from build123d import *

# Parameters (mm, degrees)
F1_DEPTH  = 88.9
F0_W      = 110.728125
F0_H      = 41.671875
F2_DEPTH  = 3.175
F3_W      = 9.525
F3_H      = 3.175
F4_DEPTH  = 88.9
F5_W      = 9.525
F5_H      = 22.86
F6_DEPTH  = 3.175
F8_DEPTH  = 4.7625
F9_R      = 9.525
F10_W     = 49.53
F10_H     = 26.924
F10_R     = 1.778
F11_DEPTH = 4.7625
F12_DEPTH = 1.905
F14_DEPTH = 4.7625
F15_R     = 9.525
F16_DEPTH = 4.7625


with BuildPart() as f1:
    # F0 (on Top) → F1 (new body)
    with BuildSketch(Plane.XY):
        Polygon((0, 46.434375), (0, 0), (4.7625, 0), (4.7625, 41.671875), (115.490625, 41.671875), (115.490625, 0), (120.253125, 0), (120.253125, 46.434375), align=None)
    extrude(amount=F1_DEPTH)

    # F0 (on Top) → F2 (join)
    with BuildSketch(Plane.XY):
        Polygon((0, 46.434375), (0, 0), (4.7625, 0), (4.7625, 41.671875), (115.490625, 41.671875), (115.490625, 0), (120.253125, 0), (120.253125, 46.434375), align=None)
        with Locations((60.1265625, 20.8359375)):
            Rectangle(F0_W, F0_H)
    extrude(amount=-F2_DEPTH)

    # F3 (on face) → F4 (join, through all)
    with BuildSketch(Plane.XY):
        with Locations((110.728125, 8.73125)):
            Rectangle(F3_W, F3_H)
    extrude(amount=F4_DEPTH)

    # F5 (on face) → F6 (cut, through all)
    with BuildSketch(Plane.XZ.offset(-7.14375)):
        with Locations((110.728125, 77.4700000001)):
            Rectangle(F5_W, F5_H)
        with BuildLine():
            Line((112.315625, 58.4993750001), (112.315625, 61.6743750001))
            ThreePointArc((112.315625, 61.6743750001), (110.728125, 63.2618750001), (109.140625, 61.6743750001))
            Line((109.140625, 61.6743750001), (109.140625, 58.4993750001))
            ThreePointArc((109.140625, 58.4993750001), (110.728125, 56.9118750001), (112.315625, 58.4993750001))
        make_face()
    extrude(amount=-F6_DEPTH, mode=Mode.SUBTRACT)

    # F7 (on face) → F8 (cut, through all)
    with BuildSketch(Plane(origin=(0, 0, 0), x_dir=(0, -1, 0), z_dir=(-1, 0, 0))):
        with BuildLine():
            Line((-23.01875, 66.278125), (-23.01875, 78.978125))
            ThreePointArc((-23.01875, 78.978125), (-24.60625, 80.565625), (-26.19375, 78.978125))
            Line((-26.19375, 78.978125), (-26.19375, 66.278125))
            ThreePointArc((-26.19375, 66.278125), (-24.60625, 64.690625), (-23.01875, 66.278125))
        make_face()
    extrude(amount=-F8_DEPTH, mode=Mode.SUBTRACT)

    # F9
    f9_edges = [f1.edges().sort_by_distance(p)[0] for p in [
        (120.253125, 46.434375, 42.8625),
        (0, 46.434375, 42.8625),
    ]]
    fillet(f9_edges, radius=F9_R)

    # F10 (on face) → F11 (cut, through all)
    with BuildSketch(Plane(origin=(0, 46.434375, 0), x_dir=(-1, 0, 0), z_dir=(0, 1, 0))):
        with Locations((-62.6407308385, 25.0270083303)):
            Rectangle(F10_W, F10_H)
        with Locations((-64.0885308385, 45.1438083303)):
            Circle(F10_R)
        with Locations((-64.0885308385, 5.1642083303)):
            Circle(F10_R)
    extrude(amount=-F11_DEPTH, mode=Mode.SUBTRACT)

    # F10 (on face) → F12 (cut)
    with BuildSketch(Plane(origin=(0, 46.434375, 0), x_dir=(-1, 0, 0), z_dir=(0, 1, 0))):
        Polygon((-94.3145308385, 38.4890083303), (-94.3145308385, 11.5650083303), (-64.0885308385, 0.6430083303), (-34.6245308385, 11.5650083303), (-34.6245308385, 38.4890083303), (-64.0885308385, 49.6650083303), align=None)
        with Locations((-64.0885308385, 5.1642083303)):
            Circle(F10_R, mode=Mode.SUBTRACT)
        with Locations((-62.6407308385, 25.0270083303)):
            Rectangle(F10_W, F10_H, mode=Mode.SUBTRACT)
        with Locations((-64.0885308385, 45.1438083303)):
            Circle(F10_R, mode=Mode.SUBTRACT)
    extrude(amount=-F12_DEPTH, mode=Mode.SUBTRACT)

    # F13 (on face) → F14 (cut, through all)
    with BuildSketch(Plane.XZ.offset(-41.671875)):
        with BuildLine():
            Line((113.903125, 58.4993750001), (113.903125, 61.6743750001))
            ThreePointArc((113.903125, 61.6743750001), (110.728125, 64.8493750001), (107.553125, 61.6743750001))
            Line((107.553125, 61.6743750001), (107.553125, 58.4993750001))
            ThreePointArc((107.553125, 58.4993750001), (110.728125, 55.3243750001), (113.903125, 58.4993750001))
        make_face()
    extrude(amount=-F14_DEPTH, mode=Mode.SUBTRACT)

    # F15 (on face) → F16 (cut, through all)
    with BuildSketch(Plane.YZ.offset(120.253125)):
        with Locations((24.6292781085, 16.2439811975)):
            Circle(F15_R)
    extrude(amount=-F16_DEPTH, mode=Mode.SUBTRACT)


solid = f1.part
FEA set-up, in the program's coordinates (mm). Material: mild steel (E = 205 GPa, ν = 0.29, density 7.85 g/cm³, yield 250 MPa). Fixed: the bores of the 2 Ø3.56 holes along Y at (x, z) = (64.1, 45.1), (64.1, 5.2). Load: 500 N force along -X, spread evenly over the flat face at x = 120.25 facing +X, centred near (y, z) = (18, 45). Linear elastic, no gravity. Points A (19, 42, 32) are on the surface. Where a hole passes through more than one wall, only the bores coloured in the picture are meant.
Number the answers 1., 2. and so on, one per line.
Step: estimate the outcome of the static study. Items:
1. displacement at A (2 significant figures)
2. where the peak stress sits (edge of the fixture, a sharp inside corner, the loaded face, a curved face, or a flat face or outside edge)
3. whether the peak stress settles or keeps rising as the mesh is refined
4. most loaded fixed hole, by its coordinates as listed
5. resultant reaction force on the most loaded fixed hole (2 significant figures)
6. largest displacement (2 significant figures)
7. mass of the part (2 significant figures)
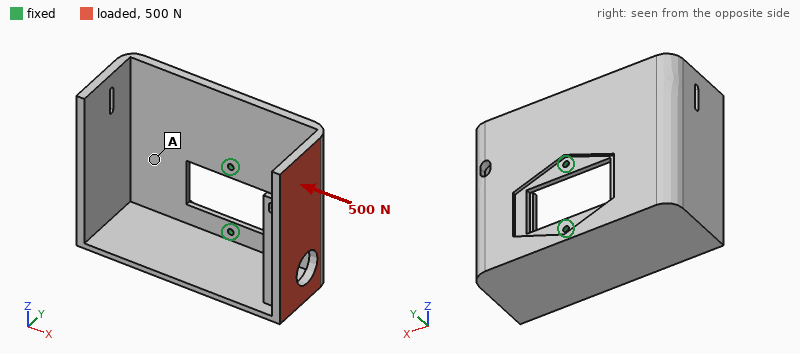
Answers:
1. 0.098 mm
2. edge of the fixture
3. keeps rising
4. (64.1, 45.1)
5. 490 N
6. 0.26 mm
7. 720 g
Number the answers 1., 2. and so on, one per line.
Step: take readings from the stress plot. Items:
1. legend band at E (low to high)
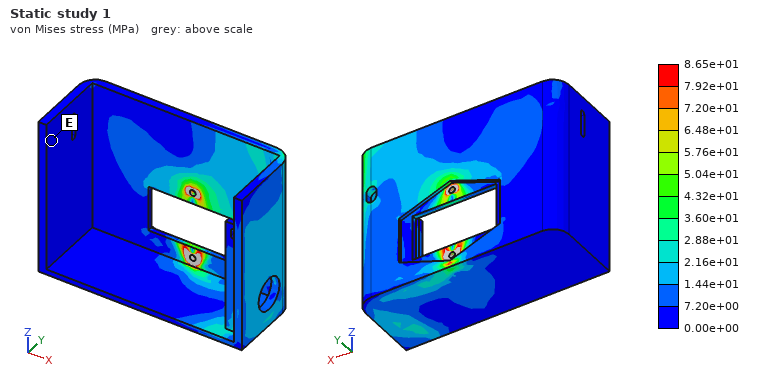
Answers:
1. 0.00e+00 to 7.20e+00 MPa
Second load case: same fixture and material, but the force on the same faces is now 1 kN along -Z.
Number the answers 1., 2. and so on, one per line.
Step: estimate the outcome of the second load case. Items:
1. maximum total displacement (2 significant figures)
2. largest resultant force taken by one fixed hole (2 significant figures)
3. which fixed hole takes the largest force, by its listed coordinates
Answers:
1. 0.26 mm
2. 1.5 kN
3. (64.1, 45.1)
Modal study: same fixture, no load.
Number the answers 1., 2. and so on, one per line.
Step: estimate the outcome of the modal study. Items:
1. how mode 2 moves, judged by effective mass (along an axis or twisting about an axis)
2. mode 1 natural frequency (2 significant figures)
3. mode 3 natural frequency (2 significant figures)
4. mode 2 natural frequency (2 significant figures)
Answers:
1. along Y
2. 280 Hz
3. 700 Hz
4. 560 Hz
